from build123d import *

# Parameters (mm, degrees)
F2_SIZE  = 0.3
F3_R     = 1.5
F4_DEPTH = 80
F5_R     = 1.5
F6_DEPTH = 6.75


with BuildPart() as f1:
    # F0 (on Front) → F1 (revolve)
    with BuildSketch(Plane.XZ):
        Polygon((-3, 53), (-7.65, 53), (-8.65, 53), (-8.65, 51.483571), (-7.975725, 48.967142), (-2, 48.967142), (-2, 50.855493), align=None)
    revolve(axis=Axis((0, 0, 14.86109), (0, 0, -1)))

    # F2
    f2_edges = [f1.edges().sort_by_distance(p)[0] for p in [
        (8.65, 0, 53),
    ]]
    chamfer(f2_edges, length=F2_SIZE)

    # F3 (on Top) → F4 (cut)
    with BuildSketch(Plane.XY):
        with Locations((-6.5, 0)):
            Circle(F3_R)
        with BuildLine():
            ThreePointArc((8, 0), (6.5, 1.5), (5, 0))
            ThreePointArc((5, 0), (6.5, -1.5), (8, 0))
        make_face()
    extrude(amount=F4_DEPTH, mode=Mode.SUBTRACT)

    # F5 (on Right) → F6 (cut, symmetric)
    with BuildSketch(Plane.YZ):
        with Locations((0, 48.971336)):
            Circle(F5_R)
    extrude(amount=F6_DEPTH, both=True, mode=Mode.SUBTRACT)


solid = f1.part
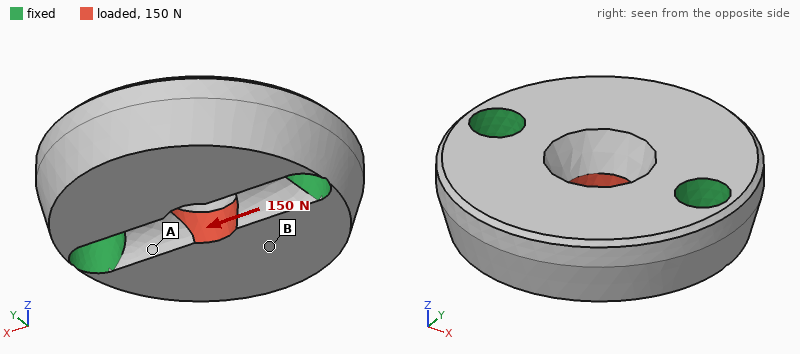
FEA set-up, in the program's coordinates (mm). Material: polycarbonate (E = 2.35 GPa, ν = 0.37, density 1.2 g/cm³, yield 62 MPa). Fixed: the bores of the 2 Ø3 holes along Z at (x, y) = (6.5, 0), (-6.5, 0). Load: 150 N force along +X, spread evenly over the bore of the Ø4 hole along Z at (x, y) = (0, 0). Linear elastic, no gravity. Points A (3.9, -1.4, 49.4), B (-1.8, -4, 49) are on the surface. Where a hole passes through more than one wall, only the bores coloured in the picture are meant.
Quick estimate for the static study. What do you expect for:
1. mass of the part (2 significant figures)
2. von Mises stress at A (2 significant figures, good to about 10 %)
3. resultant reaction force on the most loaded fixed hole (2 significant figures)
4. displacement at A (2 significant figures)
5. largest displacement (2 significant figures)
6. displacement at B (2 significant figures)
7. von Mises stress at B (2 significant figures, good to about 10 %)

0.90 g
5.4 MPa
76 N
6.1 µm
16 µm
7.5 µm
1.7 MPa
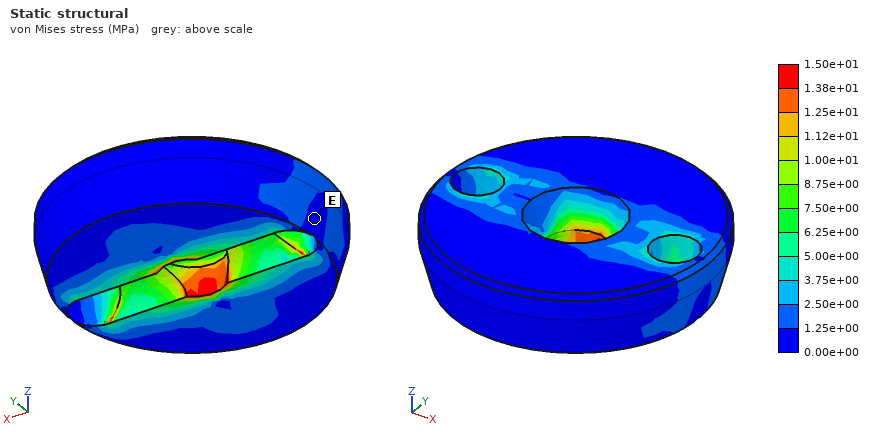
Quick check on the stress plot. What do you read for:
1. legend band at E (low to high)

0.00e+00 to 1.25e+00 MPa
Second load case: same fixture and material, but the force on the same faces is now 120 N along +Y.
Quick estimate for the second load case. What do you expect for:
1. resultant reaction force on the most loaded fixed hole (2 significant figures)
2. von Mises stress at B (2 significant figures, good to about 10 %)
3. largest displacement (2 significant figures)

60 N
4.0 MPa
22 µm
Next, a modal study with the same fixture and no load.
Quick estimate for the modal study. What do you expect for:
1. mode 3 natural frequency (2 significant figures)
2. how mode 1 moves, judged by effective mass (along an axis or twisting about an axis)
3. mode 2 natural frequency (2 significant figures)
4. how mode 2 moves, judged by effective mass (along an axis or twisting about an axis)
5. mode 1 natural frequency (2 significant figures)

26 kHz
twisting about X
12 kHz
along Z
11 kHz
